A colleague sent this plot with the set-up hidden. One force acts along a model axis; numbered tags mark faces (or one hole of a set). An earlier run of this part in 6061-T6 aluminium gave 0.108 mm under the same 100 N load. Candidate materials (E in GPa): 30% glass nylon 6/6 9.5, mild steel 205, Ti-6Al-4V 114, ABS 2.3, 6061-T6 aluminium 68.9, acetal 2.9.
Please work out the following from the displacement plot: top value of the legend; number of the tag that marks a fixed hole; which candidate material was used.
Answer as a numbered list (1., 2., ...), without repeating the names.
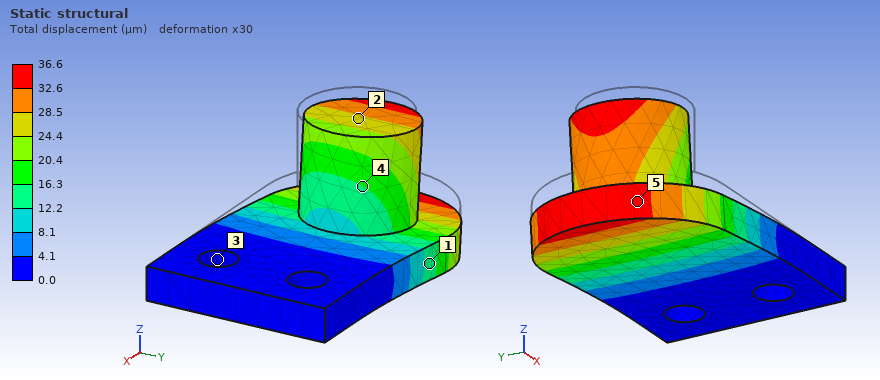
1. 36.6 µm
2. 3
3. mild steel
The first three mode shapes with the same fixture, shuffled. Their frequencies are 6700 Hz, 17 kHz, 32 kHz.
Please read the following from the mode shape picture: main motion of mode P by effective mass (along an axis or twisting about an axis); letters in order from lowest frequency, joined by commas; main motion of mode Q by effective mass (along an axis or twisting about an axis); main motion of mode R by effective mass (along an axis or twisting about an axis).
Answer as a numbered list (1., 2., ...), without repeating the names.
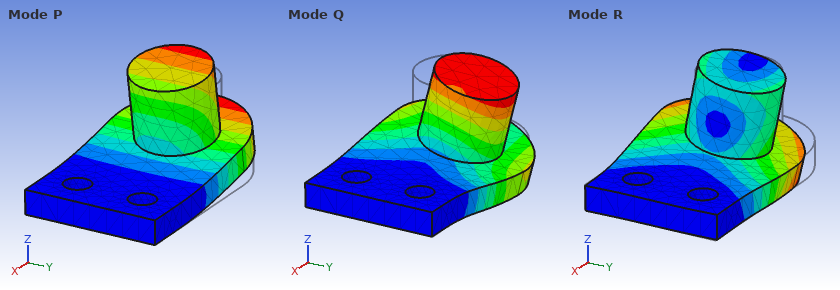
1. along Z
2. P, Q, R
3. along Y
4. along Y
